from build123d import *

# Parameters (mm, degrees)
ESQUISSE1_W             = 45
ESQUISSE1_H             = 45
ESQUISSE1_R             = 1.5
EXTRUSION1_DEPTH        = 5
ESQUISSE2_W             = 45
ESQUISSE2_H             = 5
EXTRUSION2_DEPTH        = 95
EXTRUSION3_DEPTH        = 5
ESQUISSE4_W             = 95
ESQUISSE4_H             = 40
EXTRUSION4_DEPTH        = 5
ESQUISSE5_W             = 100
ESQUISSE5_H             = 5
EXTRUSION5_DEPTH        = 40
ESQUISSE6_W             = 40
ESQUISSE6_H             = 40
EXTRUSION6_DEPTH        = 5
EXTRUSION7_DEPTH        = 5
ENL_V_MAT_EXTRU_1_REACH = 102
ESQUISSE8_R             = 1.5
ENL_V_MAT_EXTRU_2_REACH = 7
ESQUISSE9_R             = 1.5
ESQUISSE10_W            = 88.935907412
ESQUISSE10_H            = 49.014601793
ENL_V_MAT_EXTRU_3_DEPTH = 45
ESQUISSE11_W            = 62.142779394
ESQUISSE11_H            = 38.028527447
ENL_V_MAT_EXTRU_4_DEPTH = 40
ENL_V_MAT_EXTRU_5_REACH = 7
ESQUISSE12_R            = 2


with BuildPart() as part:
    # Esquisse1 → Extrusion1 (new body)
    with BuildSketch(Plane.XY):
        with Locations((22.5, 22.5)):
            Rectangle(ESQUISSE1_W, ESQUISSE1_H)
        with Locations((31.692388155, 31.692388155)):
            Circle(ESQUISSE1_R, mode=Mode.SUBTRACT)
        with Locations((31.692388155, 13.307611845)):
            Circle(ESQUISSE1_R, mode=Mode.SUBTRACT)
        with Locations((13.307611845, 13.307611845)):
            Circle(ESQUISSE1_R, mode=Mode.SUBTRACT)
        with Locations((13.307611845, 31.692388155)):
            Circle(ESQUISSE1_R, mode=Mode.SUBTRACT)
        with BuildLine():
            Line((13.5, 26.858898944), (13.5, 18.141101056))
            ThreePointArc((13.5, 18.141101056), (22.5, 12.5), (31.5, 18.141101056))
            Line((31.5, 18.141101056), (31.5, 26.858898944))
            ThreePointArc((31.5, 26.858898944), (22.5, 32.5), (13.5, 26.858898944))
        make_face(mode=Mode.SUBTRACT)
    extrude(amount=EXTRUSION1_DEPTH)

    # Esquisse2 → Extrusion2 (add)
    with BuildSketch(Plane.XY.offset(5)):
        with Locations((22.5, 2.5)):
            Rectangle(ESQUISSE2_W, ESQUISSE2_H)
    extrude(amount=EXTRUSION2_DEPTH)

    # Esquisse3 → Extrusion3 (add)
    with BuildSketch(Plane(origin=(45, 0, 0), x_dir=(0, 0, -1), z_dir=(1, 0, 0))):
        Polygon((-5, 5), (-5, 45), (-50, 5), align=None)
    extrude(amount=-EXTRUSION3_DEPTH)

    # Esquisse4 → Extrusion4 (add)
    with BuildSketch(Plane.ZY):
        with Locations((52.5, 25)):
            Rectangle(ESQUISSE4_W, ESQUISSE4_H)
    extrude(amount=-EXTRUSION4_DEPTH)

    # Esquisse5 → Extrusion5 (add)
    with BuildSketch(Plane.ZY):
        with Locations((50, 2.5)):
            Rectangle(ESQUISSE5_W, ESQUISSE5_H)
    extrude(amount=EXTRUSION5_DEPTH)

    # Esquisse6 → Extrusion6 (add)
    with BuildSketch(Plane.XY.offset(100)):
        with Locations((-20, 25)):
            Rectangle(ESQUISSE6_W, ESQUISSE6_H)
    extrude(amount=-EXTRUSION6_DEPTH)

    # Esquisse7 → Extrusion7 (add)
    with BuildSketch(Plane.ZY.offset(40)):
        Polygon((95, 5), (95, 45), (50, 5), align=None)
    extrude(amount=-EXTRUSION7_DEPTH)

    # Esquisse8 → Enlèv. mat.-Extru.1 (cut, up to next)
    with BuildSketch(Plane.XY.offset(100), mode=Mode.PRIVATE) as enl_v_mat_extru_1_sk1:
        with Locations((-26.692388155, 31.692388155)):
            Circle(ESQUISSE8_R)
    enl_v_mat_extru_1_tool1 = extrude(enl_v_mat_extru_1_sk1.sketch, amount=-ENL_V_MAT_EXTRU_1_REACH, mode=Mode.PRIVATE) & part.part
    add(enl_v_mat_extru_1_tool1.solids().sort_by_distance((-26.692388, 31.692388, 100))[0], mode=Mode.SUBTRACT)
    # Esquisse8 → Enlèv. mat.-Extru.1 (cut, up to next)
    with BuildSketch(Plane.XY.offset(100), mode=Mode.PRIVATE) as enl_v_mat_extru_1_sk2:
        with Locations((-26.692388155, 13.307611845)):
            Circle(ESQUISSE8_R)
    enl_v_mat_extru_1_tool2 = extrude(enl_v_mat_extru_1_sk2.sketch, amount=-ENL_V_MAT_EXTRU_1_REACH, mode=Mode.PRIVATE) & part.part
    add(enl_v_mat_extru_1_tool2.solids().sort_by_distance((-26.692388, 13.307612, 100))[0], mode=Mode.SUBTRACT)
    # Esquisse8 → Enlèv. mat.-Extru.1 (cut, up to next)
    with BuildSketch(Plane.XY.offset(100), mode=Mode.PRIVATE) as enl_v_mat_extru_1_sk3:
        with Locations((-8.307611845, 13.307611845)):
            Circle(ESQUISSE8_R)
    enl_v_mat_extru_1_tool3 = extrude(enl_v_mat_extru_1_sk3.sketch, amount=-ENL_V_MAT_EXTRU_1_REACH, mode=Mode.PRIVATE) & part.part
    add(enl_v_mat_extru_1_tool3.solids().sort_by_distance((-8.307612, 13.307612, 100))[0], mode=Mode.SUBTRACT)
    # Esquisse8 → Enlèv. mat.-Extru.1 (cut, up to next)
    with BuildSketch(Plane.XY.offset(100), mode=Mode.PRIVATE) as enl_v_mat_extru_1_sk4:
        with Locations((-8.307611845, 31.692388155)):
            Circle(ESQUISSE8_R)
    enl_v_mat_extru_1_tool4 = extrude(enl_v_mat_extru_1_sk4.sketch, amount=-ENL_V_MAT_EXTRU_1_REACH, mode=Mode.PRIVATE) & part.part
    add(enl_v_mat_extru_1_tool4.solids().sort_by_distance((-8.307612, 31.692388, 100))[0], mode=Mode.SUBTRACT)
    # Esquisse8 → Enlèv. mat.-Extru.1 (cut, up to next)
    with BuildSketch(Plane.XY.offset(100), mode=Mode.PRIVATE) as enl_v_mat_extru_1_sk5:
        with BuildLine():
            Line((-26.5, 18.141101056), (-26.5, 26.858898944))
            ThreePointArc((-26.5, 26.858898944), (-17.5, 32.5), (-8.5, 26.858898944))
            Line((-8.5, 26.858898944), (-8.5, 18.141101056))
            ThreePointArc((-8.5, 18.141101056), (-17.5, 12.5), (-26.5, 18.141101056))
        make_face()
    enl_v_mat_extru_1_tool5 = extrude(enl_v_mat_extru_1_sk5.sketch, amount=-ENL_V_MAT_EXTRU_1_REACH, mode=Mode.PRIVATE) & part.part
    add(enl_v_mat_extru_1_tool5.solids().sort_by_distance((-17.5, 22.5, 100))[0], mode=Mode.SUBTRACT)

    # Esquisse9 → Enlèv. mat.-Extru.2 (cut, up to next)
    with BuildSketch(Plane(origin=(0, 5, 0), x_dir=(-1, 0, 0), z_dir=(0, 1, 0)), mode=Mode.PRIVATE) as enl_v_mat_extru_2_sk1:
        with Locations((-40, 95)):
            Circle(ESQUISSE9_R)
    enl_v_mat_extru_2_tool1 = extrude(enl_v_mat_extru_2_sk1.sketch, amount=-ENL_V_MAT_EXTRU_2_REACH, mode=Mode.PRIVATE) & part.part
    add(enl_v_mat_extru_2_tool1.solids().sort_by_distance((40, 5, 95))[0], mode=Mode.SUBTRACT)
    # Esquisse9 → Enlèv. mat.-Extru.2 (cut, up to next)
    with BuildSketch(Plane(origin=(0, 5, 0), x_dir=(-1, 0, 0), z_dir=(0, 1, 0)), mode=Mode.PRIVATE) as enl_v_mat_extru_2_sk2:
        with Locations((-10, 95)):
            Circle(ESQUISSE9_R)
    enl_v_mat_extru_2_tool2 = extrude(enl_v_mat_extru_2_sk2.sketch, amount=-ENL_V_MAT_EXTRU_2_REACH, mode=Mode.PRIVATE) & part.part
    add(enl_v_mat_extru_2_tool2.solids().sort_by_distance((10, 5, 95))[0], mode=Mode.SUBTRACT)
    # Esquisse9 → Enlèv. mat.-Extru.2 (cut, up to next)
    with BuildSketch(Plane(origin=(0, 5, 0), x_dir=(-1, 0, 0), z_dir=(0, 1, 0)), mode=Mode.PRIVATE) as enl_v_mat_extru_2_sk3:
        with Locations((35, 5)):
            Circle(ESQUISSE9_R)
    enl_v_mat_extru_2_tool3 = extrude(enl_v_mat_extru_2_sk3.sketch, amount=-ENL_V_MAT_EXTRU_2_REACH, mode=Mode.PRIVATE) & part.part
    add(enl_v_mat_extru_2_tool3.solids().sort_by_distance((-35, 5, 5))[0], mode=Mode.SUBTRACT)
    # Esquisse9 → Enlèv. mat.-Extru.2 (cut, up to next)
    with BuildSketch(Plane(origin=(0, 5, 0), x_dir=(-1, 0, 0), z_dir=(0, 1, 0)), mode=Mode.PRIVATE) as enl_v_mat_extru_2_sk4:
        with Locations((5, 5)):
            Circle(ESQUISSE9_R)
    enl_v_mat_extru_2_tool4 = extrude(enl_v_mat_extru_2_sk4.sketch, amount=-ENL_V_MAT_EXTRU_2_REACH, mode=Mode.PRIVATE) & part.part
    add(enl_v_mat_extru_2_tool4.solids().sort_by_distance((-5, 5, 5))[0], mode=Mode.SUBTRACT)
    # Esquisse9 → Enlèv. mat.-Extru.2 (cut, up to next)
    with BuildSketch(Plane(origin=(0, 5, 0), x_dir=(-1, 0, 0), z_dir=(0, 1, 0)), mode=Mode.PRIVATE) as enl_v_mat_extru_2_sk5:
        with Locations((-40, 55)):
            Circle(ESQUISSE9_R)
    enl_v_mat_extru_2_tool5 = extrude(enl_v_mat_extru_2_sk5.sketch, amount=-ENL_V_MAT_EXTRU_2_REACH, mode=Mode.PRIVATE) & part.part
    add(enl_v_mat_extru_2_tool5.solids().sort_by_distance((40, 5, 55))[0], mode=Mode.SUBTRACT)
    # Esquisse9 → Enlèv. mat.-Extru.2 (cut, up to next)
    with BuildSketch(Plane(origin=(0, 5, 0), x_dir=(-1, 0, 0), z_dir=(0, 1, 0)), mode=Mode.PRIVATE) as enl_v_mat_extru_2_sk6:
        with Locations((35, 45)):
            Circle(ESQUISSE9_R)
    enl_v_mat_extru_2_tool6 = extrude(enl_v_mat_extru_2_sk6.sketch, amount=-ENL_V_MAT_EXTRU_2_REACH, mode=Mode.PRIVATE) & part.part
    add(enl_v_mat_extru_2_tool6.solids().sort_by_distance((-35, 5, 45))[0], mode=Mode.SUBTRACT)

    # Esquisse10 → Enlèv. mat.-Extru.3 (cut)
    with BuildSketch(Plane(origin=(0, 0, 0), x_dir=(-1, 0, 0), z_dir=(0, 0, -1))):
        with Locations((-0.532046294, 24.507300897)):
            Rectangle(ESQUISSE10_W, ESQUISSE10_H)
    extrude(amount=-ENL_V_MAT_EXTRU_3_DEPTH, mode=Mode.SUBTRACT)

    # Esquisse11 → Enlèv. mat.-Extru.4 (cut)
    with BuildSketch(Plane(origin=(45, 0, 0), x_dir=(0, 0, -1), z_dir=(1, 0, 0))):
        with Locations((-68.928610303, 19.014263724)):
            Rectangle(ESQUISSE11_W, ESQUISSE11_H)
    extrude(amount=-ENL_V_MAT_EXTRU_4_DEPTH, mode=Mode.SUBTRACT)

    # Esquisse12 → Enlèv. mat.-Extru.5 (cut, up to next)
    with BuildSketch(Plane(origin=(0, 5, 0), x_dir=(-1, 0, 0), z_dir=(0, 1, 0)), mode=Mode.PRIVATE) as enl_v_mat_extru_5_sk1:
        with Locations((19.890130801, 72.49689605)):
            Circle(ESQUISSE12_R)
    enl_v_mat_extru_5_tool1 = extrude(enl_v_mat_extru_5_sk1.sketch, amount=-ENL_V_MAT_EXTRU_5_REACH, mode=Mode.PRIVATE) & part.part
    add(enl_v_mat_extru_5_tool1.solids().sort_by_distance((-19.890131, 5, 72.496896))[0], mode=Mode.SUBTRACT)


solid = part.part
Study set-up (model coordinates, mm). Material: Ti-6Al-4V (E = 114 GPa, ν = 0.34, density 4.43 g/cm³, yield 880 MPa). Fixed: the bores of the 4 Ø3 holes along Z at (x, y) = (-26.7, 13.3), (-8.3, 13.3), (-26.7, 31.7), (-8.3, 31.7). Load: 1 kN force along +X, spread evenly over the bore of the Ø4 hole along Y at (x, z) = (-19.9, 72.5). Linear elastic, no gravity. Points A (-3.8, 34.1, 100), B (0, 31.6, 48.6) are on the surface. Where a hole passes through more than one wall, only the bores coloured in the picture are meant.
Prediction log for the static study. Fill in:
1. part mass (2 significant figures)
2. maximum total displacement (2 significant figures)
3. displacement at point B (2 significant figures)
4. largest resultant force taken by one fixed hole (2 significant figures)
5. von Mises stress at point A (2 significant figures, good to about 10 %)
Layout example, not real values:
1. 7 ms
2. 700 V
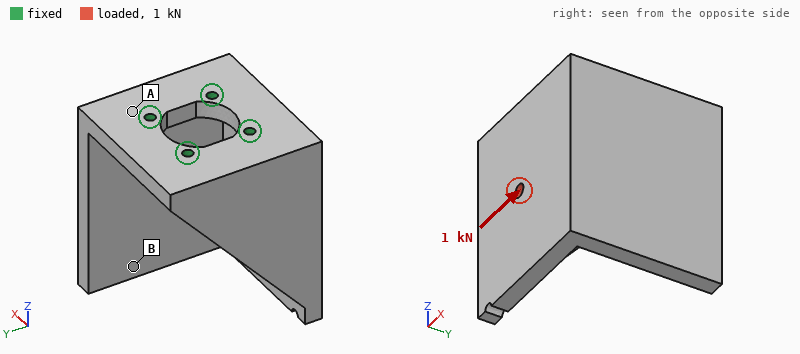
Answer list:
1. 150 g
2. 52 µm
3. 48 µm
4. 1.1 kN
5. 18 MPa
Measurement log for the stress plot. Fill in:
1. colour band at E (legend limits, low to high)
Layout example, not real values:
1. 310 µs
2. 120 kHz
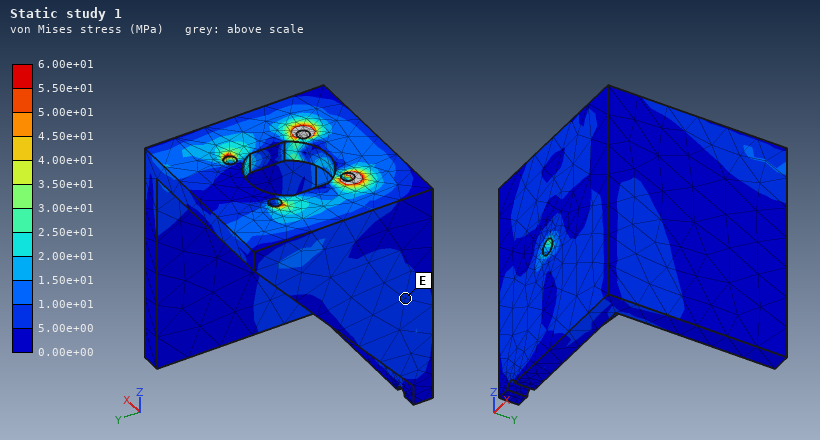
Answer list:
1. 5.00e+00 to 1.00e+01 MPa
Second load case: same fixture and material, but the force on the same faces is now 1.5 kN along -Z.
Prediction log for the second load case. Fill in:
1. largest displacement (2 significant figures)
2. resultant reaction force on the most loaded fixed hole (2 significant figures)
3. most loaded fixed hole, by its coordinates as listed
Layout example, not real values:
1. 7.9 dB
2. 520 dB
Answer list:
1. 31 µm
2. 1.1 kN
3. (-26.7, 13.3)
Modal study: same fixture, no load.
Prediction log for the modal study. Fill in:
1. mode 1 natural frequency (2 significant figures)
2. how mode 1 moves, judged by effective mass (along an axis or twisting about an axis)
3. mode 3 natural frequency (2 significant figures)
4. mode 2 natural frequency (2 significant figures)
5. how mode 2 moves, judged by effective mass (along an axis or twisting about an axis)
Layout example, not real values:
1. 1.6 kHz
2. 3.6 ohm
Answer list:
1. 2100 Hz
2. along X
3. 4300 Hz
4. 2800 Hz
5. along Y
